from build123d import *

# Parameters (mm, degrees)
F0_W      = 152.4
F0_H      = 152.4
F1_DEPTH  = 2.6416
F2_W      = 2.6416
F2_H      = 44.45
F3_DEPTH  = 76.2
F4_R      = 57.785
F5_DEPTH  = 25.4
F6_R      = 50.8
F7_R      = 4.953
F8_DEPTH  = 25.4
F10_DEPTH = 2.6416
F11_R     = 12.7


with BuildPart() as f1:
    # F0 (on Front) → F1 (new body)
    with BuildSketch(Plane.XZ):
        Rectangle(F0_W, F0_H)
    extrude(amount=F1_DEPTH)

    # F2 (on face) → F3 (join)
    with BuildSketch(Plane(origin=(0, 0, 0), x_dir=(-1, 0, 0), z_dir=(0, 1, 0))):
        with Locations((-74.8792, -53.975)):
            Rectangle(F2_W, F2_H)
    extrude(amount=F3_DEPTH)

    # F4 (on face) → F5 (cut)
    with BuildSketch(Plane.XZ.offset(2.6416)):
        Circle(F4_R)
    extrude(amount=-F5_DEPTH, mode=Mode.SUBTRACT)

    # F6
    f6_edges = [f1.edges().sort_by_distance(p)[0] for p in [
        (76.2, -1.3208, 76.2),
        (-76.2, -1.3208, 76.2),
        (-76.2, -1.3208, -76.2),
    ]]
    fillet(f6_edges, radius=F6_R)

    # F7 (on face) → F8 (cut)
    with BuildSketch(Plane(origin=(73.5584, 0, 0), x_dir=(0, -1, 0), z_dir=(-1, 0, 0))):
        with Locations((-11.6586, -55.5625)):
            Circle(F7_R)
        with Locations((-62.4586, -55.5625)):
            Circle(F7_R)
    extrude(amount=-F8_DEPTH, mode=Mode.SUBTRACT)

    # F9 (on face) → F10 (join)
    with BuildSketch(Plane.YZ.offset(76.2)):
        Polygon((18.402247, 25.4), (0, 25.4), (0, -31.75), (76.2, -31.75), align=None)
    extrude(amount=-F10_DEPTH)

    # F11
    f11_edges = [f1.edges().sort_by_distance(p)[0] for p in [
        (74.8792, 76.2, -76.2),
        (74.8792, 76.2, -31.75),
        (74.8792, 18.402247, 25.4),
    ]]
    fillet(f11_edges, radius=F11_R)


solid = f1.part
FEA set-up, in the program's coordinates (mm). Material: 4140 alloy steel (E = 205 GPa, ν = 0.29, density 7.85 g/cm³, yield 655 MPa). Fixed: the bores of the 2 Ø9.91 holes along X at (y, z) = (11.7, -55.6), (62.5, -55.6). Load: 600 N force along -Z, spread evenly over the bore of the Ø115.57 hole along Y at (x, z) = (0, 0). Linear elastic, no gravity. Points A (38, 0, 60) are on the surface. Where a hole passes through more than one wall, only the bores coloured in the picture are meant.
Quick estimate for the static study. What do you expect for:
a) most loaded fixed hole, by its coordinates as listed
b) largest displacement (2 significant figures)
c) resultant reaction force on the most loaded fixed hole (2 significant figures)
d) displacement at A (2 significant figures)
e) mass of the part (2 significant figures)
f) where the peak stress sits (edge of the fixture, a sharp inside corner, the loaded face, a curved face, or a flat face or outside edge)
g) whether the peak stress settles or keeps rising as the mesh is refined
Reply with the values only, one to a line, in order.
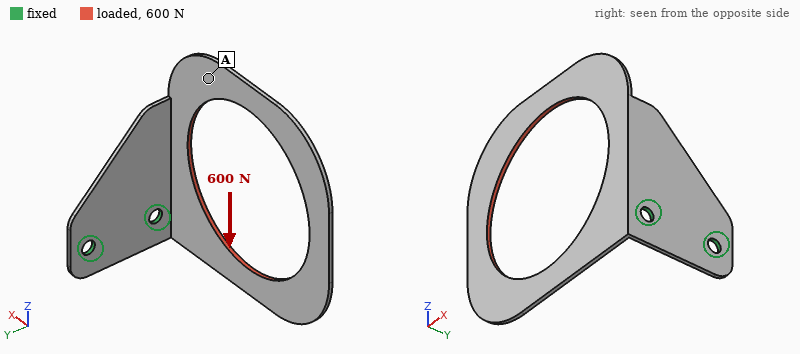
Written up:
(11.7, -55.6)
2.4 mm
650 N
1.5 mm
350 g
edge of the fixture
keeps rising
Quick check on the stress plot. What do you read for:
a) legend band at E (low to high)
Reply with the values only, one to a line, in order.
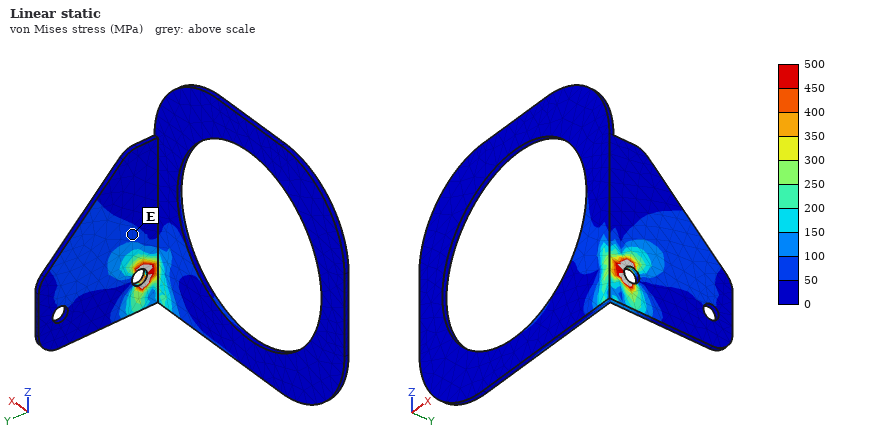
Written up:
50 to 100 MPa
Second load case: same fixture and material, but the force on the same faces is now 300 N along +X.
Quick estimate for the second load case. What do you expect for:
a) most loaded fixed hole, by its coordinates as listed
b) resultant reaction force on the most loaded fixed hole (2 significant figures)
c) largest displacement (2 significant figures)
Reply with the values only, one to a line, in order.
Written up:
(11.7, -55.6)
320 N
0.96 mm
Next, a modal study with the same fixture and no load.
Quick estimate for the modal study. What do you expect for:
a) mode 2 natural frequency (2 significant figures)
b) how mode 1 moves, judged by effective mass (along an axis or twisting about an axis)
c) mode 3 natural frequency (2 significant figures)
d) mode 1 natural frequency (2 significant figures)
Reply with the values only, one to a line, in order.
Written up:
160 Hz
along Y
180 Hz
66 Hz
